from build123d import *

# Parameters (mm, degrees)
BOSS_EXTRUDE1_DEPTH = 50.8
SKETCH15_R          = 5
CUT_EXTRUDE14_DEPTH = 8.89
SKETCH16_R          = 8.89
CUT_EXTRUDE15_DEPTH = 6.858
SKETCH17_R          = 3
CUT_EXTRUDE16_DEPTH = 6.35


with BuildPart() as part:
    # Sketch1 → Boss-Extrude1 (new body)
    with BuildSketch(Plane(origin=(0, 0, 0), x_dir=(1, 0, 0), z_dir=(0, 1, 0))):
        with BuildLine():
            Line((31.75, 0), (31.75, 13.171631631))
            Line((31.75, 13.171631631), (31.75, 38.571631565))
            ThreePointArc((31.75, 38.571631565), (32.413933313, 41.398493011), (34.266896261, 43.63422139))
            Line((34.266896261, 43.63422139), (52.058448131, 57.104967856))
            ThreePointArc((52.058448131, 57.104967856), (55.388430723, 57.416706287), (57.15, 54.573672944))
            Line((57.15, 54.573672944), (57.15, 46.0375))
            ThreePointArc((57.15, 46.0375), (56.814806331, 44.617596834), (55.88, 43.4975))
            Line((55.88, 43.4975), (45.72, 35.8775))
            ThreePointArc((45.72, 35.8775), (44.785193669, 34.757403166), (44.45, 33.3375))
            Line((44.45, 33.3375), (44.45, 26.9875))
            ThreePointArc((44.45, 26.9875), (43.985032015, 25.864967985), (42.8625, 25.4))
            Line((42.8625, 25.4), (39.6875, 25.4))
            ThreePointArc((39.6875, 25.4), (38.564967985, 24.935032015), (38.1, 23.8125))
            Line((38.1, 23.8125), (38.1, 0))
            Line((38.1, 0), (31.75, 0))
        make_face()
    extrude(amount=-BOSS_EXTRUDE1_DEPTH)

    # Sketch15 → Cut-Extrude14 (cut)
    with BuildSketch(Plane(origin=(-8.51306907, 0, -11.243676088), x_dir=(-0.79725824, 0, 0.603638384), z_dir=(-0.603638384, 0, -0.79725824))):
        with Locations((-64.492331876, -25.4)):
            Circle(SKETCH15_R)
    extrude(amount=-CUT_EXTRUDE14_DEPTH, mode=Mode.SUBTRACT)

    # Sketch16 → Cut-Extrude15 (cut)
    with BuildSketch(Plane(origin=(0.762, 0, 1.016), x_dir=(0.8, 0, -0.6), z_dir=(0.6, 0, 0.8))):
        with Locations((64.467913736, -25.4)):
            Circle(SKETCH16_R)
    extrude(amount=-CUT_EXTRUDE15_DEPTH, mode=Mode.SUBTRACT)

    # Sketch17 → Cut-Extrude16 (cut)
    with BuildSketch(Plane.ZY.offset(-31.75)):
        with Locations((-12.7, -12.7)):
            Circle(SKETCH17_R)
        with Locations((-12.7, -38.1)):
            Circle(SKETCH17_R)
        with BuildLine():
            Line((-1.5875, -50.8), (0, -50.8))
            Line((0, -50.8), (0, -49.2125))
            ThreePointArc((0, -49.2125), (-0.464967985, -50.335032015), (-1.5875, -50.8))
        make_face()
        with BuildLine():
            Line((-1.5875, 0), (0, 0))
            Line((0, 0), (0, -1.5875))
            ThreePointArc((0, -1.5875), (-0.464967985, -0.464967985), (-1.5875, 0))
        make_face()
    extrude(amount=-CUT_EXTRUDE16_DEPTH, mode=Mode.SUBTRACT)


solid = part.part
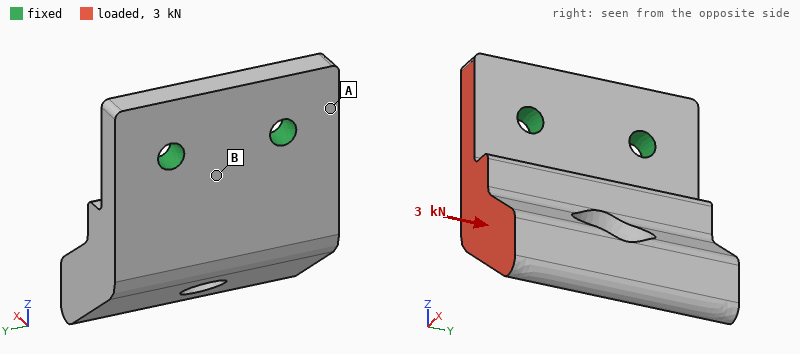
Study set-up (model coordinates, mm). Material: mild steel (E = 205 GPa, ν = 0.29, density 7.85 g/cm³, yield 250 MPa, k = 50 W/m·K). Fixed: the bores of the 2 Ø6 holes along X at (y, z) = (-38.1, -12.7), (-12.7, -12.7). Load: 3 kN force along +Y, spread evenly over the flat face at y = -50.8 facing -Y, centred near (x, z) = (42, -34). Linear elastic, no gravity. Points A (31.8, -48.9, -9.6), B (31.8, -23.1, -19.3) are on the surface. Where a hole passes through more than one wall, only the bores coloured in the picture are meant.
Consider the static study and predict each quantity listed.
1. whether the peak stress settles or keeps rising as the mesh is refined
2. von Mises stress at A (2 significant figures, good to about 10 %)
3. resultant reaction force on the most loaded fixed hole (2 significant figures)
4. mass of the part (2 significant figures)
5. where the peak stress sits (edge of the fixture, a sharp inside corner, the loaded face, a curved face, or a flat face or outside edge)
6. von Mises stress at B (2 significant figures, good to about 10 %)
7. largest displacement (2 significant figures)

keeps rising
22 MPa
2.8 kN
230 g
edge of the fixture
8.1 MPa
14 µm
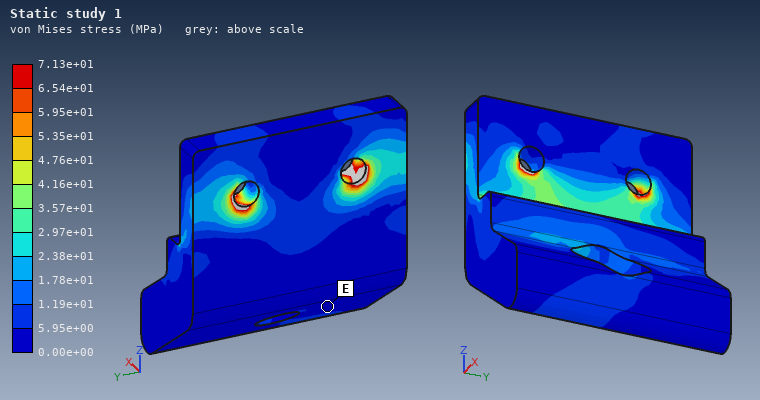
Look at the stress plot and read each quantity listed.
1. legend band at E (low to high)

0.00e+00 to 5.95e+00 MPa
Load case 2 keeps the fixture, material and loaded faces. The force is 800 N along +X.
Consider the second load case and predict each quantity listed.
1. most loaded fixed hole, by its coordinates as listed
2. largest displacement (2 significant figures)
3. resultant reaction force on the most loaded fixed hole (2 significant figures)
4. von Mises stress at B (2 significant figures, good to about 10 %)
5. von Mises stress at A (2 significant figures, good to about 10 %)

(-38.1, -12.7)
45 µm
990 N
30 MPa
17 MPa
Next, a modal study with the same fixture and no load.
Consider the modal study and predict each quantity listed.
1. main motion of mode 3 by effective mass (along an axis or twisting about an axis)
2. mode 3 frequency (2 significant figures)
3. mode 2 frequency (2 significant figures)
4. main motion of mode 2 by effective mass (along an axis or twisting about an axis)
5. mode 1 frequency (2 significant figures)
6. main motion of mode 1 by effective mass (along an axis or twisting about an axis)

along Y
8200 Hz
5000 Hz
along Y
1900 Hz
along X
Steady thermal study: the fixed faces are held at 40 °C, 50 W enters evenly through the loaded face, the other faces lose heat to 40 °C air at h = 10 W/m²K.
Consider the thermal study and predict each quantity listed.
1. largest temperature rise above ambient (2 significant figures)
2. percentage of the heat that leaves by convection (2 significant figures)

86 K
5.9 %
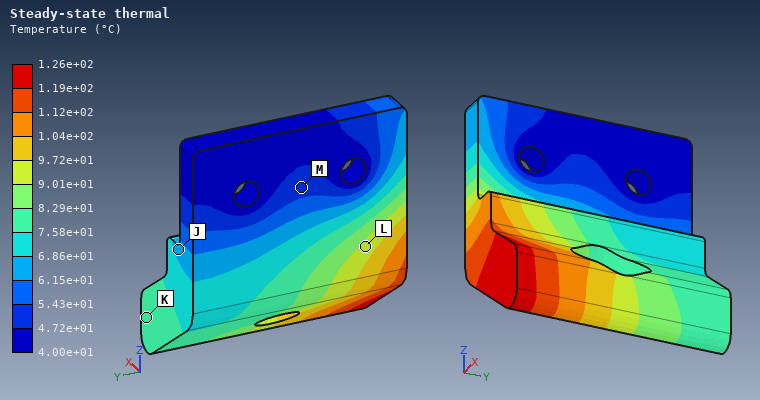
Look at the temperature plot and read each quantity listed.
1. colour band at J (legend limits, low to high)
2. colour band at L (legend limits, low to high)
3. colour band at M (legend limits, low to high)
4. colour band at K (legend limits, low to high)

6.15e+01 to 6.86e+01 °C
9.01e+01 to 9.72e+01 °C
4.72e+01 to 5.43e+01 °C
7.58e+01 to 8.29e+01 °C
